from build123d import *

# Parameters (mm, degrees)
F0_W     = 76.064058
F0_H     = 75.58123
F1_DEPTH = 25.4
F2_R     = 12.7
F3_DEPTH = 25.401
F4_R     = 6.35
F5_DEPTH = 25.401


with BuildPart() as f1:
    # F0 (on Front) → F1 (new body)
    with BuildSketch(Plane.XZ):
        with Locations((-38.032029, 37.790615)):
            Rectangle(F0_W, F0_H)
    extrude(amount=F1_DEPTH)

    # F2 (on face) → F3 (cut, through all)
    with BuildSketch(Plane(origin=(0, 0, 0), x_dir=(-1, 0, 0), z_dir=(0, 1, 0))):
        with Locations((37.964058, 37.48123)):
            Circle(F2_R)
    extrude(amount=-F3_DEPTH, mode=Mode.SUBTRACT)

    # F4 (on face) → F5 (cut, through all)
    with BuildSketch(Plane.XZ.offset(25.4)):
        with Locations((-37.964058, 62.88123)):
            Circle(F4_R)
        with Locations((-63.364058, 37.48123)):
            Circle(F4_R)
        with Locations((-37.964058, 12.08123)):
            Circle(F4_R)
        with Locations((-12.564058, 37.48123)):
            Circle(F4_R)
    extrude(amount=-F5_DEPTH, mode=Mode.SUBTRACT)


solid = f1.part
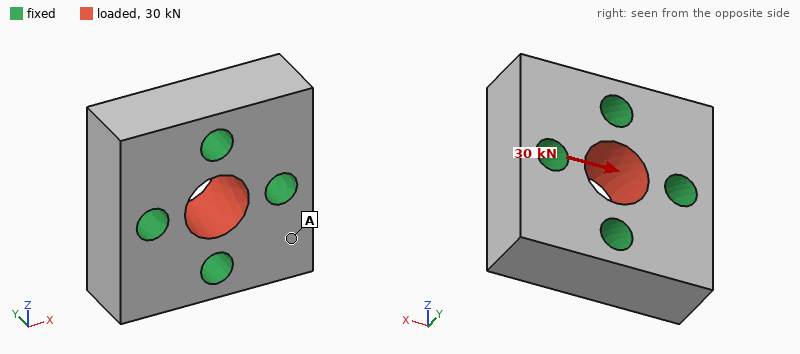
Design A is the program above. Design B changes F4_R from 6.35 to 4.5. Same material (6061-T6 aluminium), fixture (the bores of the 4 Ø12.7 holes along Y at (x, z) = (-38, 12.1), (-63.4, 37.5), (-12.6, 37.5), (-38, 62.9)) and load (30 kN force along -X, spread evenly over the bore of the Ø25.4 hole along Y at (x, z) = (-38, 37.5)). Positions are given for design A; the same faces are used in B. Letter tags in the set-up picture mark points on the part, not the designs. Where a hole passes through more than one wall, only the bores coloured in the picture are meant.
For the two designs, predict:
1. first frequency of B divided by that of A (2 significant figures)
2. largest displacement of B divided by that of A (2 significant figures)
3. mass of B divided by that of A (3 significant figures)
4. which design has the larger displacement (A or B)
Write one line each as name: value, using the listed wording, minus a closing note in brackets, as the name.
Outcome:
first frequency of B divided by that of A: 0.88
largest displacement of B divided by that of A: 1.2
mass of B divided by that of A: 1.05
which design has the larger displacement: B
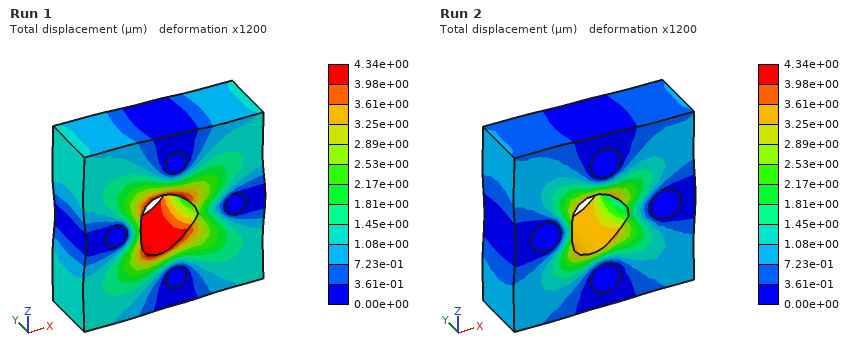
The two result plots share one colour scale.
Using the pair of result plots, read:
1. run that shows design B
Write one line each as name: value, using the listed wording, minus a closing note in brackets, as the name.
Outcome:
run that shows design B: Run 1
